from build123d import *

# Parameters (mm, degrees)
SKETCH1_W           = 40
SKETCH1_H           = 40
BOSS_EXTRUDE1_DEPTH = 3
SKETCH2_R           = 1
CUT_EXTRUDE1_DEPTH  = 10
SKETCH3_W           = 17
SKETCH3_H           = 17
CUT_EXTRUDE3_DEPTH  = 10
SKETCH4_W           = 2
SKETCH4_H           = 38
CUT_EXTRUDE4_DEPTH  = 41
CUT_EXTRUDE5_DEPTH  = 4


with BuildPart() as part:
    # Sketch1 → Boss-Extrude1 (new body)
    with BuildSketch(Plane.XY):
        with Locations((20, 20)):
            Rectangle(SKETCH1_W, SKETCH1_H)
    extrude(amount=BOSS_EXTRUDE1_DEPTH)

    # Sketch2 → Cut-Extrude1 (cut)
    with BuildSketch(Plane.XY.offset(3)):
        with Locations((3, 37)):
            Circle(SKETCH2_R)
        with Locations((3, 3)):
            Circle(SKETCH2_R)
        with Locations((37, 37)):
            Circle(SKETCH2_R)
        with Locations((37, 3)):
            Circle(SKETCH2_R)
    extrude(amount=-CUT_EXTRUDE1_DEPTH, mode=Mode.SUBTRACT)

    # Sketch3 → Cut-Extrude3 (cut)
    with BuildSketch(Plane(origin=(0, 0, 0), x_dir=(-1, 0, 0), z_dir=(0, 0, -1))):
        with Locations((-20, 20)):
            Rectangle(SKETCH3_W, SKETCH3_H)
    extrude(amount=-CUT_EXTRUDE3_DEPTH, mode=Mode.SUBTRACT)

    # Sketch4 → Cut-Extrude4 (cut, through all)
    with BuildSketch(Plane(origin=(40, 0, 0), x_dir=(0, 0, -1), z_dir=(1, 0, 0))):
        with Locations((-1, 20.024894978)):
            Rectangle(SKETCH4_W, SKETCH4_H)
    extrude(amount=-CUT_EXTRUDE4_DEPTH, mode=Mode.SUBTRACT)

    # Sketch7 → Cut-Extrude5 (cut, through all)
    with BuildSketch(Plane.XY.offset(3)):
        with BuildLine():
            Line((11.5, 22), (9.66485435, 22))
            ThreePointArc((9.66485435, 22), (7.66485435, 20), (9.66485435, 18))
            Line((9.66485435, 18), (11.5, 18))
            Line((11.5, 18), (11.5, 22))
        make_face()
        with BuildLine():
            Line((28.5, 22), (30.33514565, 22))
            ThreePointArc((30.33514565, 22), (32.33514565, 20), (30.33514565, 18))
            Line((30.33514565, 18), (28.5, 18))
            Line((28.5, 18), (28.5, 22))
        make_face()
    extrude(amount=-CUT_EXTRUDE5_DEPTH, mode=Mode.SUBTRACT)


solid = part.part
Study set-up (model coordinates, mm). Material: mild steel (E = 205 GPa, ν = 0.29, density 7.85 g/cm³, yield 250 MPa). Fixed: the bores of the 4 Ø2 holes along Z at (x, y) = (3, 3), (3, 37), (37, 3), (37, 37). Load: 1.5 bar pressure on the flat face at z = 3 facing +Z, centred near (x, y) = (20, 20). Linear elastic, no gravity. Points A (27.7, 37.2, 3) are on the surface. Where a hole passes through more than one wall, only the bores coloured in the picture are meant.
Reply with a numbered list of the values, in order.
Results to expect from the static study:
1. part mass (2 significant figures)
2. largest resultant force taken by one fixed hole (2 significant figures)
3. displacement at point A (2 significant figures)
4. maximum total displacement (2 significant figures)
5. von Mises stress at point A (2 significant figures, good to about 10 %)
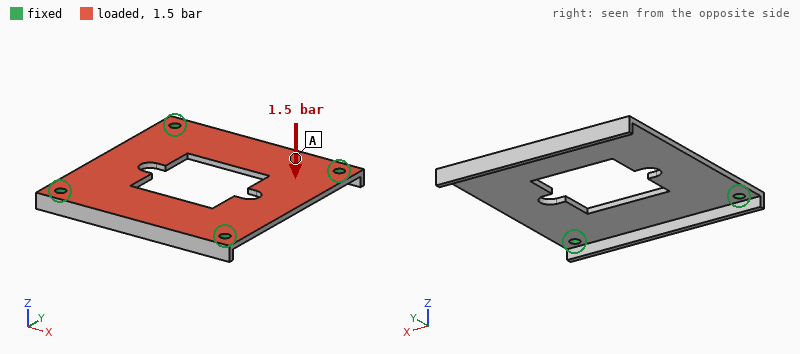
1. 11 g
2. 50 N
3. 10 µm
4. 56 µm
5. 29 MPa
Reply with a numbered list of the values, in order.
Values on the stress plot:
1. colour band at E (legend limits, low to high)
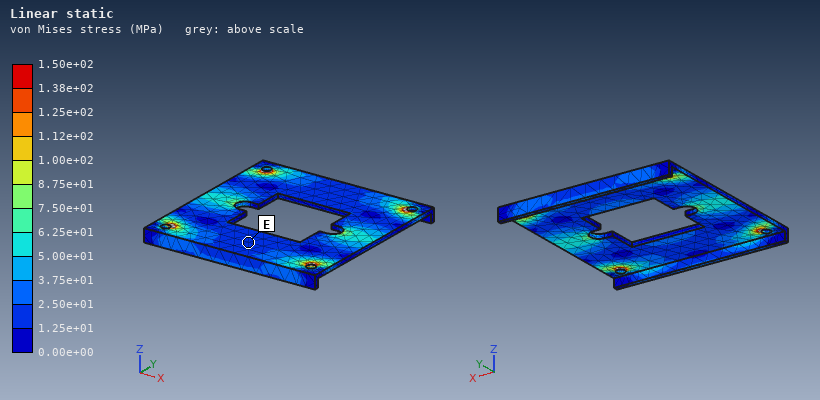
1. 1.25e+01 to 2.50e+01 MPa
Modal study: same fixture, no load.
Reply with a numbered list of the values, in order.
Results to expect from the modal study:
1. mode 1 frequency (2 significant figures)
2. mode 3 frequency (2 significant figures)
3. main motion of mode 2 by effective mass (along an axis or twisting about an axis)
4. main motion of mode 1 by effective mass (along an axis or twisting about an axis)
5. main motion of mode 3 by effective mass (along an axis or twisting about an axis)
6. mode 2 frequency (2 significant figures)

1. 3900 Hz
2. 6200 Hz
3. twisting about Y
4. along Z
5. twisting about X
6. 5000 Hz
